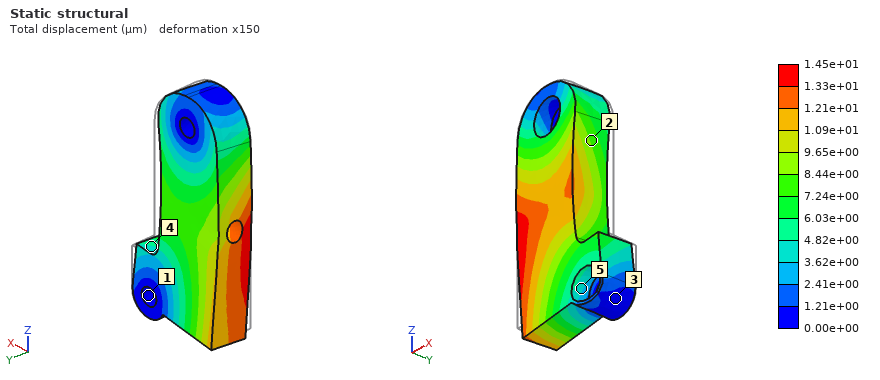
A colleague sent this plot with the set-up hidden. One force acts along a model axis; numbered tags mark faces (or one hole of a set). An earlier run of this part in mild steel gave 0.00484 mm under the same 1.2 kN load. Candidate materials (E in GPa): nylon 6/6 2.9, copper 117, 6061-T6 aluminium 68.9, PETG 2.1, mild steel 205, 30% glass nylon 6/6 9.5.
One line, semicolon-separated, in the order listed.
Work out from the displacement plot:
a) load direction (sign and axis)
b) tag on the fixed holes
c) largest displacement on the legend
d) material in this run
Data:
-X; 1; 1.45e+01 µm; 6061-T6 aluminium
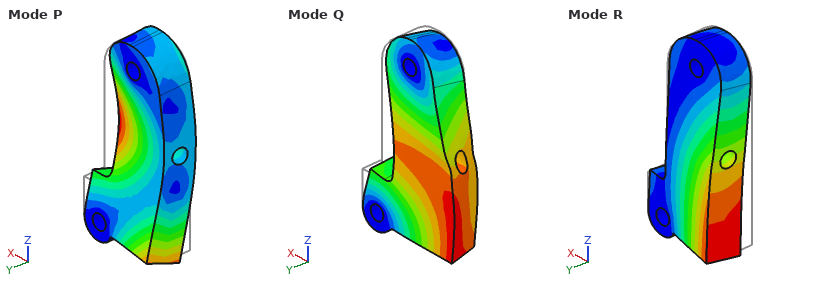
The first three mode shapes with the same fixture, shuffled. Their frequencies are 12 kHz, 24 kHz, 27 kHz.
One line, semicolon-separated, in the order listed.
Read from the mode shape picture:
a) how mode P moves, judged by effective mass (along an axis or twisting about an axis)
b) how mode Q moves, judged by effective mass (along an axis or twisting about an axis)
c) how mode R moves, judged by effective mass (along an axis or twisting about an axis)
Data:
along Y; along X; along Y
